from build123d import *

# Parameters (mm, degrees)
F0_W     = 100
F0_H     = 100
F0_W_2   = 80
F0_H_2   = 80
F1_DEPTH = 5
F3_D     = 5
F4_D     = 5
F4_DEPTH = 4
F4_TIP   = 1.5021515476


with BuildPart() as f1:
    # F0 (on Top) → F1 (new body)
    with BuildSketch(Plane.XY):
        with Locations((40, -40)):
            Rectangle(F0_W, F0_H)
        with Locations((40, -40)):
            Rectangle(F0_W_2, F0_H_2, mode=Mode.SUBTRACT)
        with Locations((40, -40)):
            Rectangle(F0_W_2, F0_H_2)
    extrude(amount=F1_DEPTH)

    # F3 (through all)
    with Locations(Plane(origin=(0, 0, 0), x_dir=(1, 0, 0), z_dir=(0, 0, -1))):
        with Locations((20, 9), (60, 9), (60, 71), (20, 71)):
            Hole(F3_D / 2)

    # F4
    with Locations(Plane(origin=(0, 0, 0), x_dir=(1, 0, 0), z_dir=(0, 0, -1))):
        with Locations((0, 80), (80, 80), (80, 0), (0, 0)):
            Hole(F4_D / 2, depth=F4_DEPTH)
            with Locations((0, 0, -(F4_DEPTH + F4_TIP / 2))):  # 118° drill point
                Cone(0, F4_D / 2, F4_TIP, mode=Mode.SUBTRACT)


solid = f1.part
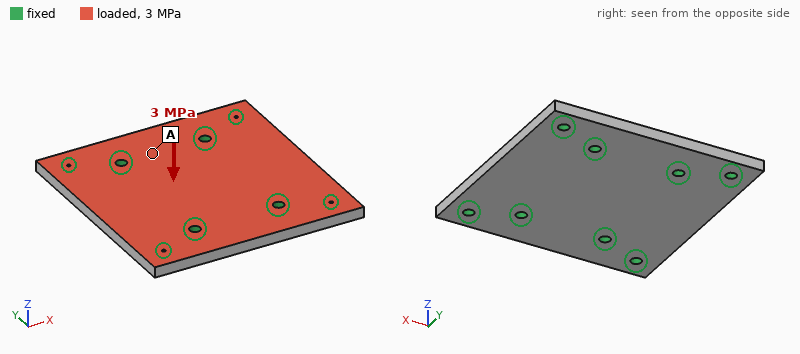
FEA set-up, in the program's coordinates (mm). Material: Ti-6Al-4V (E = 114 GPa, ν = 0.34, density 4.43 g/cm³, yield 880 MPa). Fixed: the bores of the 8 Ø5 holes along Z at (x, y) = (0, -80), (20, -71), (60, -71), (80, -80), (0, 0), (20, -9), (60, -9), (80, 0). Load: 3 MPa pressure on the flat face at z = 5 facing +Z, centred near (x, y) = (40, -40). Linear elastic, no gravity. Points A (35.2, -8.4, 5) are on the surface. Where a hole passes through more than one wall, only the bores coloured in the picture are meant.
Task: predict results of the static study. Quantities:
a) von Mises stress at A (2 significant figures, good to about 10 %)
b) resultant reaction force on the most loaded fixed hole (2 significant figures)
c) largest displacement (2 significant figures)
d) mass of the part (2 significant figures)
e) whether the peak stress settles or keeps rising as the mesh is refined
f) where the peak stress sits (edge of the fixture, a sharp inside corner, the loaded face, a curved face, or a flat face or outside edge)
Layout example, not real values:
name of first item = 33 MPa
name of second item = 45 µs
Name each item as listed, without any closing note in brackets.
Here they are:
von Mises stress at A = 88 MPa
resultant reaction force on the most loaded fixed hole = 5.2 kN
largest displacement = 0.22 mm
mass of the part = 220 g
whether the peak stress settles or keeps rising as the mesh is refined = keeps rising
where the peak stress sits = edge of the fixture
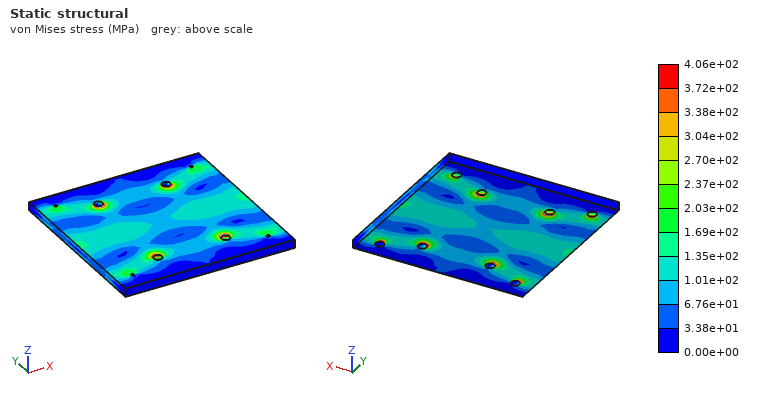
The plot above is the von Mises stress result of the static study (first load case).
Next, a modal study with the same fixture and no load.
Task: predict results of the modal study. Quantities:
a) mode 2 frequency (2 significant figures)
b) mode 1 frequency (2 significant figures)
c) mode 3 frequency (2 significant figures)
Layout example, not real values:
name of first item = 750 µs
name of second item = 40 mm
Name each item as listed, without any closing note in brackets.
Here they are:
mode 2 frequency = 5200 Hz
mode 1 frequency = 5100 Hz
mode 3 frequency = 7200 Hz
